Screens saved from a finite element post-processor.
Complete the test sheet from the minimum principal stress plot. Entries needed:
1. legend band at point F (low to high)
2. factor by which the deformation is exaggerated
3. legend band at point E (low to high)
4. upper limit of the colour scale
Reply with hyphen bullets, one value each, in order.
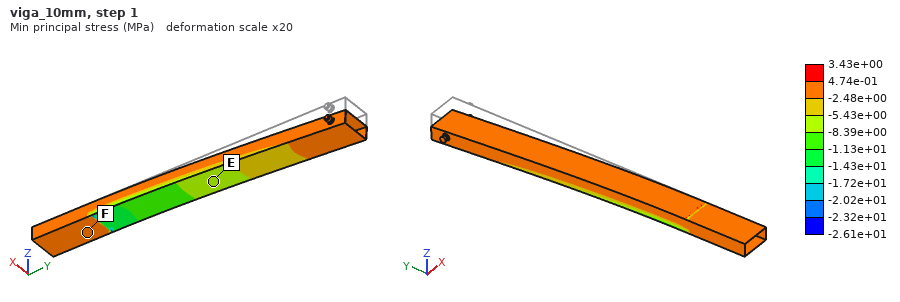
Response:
- -2.48e+00 to 4.74e-01 MPa
- 20
- -8.39e+00 to -5.43e+00 MPa
- 3.43e+00 MPa
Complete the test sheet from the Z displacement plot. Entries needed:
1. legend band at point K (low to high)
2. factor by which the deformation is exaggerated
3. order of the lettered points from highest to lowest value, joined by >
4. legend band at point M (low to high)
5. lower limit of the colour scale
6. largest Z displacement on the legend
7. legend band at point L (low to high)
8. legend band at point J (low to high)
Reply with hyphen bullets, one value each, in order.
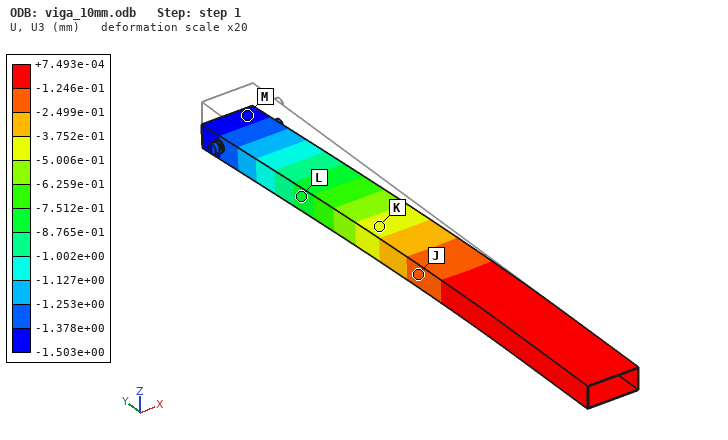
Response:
- -5.006e-01 to -3.752e-01 mm
- 20
- J > K > L > M
- -1.503e+00 to -1.378e+00 mm
- -1.503e+00 mm
- +7.493e-04 mm
- -8.765e-01 to -7.512e-01 mm
- -2.499e-01 to -1.246e-01 mm
